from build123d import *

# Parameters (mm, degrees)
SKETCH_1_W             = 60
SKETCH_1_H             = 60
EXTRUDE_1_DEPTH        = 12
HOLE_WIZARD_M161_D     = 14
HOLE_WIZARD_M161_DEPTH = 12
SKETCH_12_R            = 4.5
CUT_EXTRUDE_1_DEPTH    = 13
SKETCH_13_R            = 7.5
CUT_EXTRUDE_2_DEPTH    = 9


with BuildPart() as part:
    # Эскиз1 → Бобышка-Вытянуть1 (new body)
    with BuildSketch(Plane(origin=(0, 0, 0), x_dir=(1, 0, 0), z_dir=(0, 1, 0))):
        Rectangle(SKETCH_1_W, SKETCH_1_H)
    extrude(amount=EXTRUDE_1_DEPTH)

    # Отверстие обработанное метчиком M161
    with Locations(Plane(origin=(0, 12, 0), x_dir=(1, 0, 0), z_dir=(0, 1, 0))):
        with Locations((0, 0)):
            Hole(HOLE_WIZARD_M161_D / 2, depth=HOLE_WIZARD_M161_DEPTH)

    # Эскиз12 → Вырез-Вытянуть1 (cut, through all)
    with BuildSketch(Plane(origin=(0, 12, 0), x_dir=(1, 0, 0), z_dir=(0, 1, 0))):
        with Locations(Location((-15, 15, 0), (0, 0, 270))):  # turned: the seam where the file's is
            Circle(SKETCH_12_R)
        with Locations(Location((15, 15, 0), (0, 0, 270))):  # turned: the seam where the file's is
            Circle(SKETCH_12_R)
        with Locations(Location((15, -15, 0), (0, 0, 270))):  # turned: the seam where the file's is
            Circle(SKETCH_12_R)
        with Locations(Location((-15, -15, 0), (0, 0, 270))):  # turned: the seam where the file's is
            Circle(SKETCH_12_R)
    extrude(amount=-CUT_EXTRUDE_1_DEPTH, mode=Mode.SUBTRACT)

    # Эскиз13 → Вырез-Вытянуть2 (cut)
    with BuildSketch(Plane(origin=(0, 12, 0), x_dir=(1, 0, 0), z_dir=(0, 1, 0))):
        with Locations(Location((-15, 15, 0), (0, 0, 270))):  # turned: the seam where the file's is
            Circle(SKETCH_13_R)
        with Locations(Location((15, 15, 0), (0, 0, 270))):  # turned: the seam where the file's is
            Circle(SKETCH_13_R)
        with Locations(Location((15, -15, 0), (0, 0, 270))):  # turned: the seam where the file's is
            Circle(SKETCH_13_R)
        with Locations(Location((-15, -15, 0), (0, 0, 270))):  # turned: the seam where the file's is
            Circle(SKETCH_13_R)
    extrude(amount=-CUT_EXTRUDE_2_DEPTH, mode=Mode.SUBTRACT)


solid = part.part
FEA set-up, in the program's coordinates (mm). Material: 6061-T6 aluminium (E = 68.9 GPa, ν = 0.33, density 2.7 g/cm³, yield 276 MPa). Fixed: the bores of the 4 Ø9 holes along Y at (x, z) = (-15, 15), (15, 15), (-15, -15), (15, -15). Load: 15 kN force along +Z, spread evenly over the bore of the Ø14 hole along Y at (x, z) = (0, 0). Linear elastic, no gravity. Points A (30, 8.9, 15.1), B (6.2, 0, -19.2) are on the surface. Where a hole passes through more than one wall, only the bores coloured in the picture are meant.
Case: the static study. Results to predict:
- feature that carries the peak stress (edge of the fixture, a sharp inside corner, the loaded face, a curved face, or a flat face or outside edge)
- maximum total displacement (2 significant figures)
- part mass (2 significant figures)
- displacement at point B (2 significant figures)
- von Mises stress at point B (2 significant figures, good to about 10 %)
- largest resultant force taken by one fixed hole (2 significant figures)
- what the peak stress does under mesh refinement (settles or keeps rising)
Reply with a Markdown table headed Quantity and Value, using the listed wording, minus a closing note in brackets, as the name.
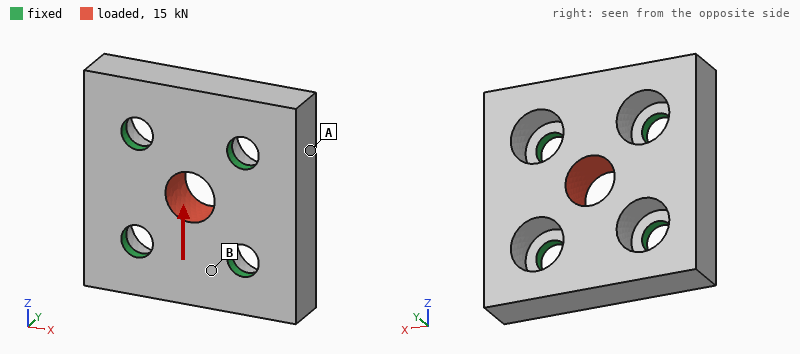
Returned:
| Quantity | Value |
|---|---|
| feature that carries the peak stress | edge of the fixture |
| maximum total displacement | 18 µm |
| part mass | 92 g |
| displacement at point B | 6.5 µm |
| von Mises stress at point B | 32 MPa |
| largest resultant force taken by one fixed hole | 4.0 kN |
| what the peak stress does under mesh refinement | keeps rising |
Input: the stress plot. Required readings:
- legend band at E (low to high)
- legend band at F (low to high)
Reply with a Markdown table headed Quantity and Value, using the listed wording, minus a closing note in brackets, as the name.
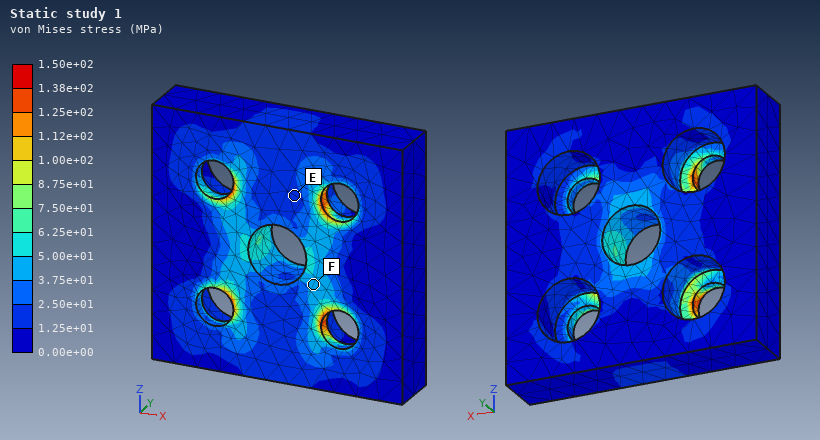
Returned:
| Quantity | Value |
|---|---|
| legend band at E | 1.25e+01 to 2.50e+01 MPa |
| legend band at F | 3.75e+01 to 5.00e+01 MPa |
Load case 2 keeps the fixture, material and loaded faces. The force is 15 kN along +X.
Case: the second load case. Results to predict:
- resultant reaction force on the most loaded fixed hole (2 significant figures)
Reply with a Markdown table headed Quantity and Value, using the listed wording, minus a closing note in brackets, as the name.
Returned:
| Quantity | Value |
|---|---|
| resultant reaction force on the most loaded fixed hole | 4.0 kN |
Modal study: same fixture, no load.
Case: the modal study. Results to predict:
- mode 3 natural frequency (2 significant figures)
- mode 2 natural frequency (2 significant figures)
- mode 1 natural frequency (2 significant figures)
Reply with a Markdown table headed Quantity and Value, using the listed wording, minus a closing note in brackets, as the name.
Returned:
| Quantity | Value |
|---|---|
| mode 3 natural frequency | 16 kHz |
| mode 2 natural frequency | 15 kHz |
| mode 1 natural frequency | 15 kHz |
